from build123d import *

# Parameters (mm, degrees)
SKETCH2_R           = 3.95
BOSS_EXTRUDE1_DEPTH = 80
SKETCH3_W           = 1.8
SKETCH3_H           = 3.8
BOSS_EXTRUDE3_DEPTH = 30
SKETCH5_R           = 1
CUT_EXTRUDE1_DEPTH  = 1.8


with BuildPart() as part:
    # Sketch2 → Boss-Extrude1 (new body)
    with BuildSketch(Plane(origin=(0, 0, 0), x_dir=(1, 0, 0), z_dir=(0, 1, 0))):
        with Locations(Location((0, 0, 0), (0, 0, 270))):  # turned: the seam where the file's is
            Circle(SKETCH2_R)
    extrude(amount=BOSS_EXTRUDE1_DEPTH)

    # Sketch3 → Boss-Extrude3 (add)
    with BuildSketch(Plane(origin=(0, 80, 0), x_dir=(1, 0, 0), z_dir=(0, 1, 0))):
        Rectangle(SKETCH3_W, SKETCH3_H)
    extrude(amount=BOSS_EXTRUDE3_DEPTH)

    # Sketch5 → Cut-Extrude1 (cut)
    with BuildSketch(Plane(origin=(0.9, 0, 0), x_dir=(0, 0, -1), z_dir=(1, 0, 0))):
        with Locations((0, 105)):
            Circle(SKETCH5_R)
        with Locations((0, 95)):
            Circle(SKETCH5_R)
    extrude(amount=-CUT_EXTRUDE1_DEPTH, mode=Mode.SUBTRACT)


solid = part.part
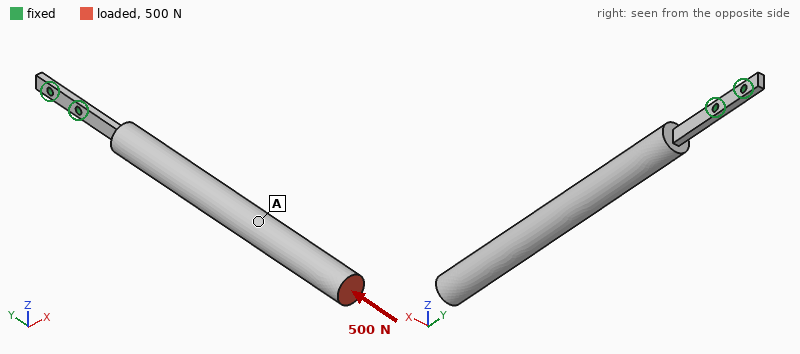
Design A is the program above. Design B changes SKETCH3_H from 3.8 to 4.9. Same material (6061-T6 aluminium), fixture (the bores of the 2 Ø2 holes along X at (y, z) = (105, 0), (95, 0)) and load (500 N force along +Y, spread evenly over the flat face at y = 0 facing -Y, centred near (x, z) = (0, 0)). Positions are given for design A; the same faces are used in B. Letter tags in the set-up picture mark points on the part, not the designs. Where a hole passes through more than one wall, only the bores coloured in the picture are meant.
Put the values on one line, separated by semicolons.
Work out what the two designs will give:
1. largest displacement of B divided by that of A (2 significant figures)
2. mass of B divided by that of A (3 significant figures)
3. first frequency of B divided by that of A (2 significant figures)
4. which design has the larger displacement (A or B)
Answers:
0.88; 1.01; 1.1; A
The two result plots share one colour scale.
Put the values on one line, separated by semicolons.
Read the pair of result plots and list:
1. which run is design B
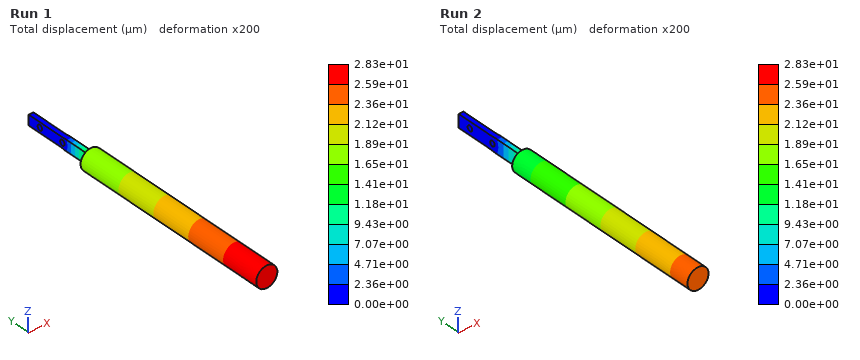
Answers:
Run 2
